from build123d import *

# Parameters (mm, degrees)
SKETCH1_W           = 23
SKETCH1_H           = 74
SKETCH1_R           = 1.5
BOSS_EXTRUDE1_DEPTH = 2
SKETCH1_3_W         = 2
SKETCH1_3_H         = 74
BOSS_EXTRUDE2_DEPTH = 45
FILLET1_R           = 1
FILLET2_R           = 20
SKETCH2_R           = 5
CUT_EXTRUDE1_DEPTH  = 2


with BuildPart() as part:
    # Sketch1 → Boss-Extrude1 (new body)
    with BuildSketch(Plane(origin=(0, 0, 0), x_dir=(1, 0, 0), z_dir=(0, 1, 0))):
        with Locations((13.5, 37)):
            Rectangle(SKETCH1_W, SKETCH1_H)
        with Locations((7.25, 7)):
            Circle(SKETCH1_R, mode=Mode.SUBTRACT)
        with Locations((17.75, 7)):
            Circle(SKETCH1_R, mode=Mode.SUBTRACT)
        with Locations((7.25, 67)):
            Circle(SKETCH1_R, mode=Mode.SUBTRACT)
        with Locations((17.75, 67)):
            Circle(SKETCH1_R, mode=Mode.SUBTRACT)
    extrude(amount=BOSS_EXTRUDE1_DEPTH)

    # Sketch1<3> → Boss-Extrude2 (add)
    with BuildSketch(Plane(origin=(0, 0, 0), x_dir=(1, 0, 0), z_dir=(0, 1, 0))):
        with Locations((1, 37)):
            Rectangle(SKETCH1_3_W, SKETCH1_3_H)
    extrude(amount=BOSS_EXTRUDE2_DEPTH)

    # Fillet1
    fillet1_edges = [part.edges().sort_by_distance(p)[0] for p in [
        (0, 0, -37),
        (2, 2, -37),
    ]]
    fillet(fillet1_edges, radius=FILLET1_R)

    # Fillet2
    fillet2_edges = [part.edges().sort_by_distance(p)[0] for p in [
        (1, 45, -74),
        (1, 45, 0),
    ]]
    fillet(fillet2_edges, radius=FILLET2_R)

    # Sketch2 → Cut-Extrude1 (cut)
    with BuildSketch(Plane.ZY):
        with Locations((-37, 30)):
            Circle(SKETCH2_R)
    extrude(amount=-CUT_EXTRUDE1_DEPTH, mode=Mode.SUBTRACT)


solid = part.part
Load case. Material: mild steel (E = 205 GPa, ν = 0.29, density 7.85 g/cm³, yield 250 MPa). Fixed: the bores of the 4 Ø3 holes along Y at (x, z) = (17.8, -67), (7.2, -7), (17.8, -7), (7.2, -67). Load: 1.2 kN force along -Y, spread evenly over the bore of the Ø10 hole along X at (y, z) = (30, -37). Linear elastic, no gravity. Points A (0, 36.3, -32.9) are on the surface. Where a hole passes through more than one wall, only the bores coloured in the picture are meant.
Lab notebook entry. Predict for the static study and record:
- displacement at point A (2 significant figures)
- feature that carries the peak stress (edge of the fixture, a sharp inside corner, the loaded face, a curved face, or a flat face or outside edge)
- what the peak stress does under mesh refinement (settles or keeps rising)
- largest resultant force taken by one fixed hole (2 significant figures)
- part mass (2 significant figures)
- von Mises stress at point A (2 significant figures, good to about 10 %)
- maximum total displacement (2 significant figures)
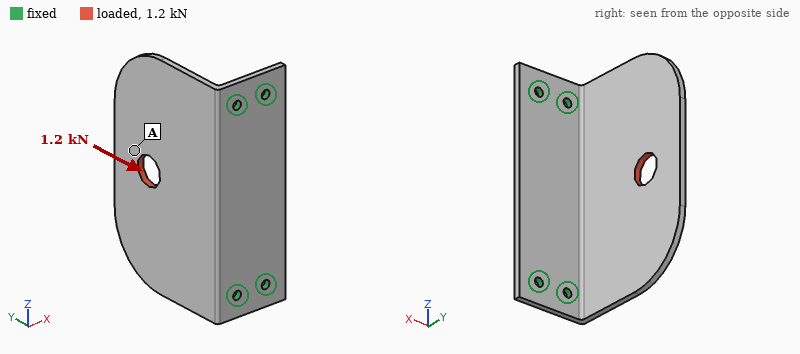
0.11 mm
edge of the fixture
keeps rising
750 N
75 g
27 MPa
0.14 mm
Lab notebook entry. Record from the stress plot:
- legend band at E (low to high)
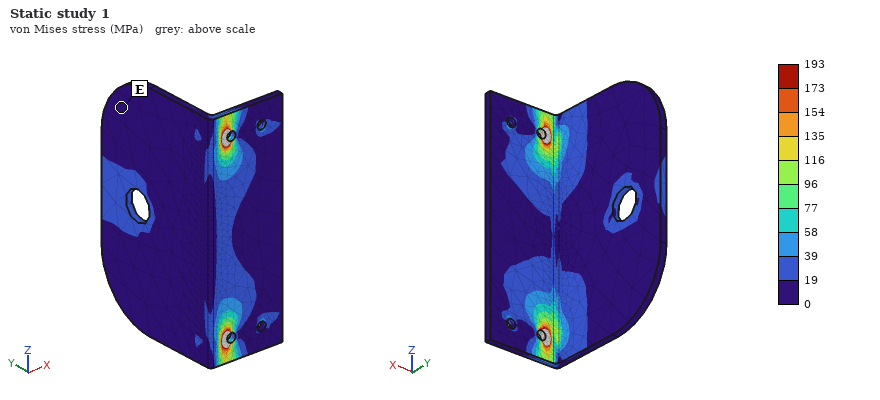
0 to 19 MPa
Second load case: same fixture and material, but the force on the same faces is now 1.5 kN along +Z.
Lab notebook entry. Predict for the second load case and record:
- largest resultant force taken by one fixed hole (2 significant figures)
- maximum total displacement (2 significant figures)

990 N
83 µm
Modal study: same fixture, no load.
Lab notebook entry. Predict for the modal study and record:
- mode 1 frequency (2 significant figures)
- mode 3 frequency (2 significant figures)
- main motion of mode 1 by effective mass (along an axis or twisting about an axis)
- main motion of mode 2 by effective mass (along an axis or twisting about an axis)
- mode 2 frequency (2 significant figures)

730 Hz
3300 Hz
along X
twisting about Y
1500 Hz
